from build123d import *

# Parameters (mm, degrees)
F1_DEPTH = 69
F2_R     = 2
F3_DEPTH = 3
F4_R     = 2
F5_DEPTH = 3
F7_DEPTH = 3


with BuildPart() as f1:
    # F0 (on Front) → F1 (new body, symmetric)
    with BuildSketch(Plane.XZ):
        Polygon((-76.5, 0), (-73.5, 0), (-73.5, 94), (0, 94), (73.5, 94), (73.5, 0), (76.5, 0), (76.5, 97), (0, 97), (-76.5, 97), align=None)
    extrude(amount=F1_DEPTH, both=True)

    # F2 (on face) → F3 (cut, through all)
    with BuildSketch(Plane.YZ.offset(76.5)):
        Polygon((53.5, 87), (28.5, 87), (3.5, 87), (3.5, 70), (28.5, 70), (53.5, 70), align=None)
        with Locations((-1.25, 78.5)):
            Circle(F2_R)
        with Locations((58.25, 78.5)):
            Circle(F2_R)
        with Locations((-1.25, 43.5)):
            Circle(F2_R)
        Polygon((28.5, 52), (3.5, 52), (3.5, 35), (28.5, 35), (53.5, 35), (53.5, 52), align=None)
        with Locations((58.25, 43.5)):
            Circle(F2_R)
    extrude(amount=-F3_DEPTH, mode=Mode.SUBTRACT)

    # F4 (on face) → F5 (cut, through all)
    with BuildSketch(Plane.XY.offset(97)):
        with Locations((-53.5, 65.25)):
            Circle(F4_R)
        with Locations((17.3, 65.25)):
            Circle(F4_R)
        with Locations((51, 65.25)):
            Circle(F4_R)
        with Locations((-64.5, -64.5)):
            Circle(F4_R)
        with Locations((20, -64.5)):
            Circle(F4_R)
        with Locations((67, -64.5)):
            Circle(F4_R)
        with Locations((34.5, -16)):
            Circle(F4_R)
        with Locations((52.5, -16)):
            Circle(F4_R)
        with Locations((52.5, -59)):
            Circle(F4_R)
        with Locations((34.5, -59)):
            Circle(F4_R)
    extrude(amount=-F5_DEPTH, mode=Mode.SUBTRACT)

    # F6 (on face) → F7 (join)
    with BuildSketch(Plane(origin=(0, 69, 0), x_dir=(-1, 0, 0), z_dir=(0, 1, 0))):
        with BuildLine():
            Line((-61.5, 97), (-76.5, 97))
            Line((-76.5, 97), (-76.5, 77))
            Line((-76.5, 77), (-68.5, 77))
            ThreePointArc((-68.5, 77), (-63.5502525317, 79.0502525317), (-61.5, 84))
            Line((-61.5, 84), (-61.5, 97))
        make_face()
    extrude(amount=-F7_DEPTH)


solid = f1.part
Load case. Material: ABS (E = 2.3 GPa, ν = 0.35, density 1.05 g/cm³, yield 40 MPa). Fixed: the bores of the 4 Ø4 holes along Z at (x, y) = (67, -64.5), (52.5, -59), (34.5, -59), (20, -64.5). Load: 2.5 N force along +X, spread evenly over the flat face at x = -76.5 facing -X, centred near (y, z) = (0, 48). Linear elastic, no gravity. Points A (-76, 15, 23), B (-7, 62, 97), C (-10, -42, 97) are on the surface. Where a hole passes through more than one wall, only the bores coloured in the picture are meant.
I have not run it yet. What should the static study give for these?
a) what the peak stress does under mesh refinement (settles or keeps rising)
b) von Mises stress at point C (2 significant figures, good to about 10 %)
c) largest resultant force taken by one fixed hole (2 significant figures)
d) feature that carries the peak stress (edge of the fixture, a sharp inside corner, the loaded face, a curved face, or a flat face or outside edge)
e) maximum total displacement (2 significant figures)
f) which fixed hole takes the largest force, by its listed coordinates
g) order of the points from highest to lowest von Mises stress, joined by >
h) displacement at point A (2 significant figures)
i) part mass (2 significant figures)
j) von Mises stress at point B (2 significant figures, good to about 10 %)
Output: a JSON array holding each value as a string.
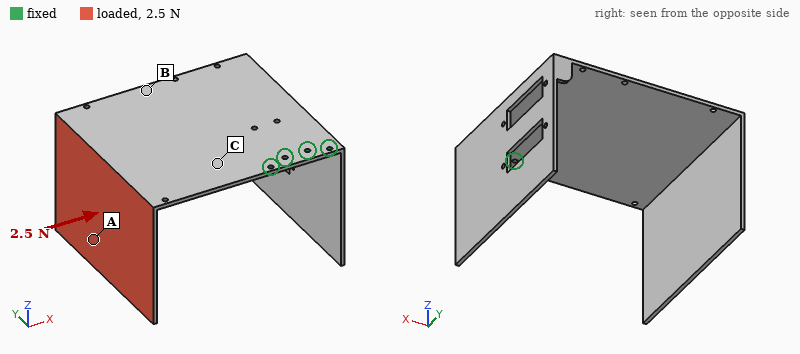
["keeps rising", "0.63 MPa", "3.7 N", "edge of the fixture", "2.7 mm", "(20, -64.5)", "C > B > A", "2.1 mm", "140 g", "0.45 MPa"]
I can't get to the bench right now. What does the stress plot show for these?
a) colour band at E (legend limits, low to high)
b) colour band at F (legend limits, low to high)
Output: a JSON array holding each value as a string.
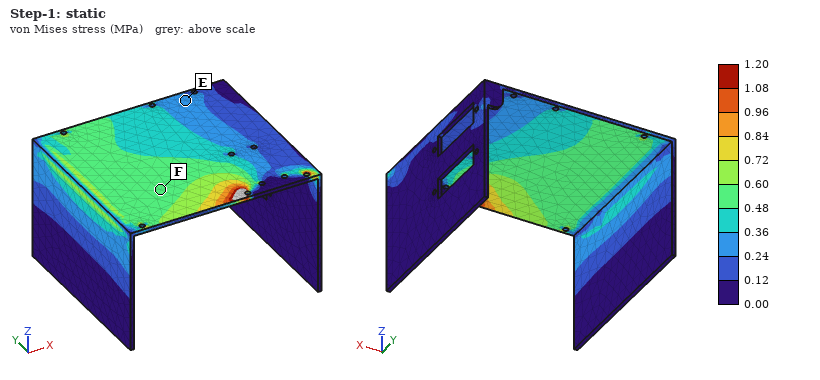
["0.24 to 0.36 MPa", "0.48 to 0.60 MPa"]
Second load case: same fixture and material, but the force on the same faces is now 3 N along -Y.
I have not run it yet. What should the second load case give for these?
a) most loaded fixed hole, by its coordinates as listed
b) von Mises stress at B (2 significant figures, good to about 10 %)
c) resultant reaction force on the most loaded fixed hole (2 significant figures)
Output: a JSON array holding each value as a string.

["(20, -64.5)", "0.43 MPa", "8.5 N"]
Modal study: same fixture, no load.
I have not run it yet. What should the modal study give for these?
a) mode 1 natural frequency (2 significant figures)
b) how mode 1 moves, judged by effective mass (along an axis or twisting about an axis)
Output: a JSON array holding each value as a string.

["18 Hz", "along Z"]
